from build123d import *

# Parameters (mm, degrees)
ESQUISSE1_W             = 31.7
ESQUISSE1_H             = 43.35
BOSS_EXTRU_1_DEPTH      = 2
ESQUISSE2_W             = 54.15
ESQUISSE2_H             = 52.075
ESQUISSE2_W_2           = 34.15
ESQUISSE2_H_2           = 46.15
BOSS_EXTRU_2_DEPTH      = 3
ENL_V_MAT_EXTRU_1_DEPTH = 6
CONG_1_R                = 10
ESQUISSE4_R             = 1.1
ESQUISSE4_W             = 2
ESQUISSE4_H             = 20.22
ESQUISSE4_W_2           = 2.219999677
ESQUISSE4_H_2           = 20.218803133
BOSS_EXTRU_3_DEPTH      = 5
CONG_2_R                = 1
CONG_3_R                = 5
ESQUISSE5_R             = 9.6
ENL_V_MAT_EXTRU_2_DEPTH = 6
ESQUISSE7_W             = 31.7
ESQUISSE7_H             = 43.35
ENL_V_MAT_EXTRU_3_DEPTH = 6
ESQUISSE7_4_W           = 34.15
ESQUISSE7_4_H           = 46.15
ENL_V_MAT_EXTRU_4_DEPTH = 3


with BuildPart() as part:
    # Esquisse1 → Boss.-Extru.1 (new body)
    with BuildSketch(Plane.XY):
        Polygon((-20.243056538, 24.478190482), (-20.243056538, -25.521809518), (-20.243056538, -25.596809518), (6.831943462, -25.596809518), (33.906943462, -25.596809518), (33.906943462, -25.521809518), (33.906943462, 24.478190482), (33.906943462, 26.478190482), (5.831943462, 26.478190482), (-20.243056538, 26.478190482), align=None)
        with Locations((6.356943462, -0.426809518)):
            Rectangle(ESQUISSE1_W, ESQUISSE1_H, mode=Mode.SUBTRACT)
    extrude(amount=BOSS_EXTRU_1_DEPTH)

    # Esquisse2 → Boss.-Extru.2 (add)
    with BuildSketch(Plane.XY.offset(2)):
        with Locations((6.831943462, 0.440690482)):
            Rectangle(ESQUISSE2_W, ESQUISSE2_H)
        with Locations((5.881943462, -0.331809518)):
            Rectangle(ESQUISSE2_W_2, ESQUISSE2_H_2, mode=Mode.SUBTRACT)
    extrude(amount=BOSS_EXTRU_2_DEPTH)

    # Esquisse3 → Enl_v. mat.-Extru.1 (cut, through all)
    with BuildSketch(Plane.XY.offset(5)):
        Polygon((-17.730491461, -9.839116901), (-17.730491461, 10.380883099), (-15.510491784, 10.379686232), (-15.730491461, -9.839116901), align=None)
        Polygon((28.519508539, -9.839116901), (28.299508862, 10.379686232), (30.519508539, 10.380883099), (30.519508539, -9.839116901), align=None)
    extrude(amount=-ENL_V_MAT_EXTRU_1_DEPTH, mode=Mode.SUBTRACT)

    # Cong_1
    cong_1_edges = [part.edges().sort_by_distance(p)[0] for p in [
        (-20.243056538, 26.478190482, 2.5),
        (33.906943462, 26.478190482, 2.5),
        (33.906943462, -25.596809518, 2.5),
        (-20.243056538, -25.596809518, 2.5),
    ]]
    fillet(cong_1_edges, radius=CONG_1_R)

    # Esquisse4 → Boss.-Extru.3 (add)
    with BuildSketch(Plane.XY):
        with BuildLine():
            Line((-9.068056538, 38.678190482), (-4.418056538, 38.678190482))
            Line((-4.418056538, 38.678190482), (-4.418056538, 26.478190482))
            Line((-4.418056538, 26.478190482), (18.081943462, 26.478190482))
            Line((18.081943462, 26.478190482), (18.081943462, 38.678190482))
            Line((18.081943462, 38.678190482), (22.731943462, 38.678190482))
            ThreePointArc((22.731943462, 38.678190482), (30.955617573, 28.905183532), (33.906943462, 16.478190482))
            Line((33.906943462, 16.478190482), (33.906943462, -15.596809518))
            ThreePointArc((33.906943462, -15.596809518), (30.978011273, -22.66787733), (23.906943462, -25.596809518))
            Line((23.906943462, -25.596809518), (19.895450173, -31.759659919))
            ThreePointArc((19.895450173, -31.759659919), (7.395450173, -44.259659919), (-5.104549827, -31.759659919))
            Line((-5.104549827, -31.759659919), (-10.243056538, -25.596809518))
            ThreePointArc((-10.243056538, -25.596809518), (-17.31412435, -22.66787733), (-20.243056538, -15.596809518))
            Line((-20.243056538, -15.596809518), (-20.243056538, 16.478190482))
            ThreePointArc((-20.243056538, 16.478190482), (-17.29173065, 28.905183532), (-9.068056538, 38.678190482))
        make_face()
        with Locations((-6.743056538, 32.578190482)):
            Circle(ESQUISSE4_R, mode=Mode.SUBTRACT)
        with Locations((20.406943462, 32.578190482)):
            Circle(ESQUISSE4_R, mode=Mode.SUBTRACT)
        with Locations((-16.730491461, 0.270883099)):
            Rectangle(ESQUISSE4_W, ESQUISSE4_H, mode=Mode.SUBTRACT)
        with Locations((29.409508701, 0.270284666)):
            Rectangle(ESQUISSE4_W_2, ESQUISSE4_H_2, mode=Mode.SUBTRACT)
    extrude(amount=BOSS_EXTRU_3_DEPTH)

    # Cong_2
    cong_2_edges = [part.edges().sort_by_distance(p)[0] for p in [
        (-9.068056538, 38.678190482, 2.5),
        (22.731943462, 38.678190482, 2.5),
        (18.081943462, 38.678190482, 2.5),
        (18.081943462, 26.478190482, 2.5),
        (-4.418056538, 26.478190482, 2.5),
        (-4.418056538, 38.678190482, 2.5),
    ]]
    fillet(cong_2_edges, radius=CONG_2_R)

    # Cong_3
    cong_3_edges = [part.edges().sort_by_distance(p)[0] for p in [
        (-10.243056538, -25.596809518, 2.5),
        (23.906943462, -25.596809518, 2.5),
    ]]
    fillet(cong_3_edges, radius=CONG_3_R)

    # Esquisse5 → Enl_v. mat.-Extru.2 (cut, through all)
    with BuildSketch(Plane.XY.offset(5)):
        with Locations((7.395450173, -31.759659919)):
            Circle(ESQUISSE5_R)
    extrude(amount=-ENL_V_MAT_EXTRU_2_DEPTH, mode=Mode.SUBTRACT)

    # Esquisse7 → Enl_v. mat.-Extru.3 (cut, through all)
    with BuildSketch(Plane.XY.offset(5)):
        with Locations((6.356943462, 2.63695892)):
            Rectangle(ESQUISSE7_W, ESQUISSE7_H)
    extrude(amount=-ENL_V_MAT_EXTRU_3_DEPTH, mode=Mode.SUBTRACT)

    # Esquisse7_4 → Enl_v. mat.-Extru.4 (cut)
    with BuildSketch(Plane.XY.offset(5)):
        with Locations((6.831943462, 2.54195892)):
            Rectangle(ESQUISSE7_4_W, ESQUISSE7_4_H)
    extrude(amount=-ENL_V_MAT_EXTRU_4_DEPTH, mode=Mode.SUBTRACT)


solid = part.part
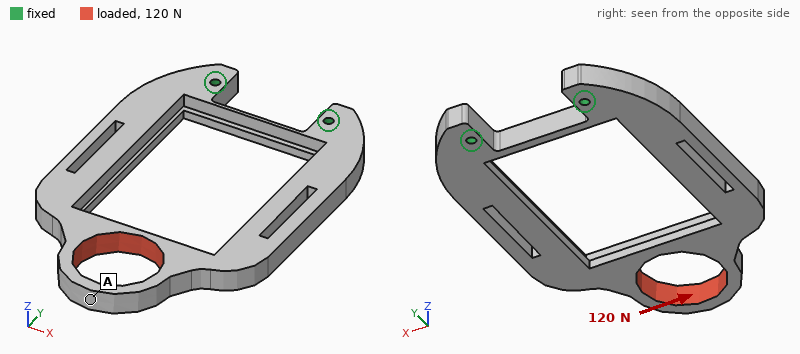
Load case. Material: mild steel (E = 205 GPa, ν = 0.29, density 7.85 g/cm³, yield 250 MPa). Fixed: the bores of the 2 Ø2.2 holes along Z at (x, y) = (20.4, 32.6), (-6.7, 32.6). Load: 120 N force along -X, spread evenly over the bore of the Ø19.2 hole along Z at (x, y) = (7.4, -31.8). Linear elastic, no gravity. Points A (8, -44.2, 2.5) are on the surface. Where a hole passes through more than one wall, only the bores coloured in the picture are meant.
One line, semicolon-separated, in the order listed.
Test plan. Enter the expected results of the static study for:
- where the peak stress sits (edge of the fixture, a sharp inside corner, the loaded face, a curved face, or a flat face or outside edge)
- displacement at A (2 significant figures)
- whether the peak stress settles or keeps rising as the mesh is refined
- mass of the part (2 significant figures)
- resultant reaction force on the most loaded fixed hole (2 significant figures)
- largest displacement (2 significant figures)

edge of the fixture; 50 µm; keeps rising; 62 g; 120 N; 51 µm
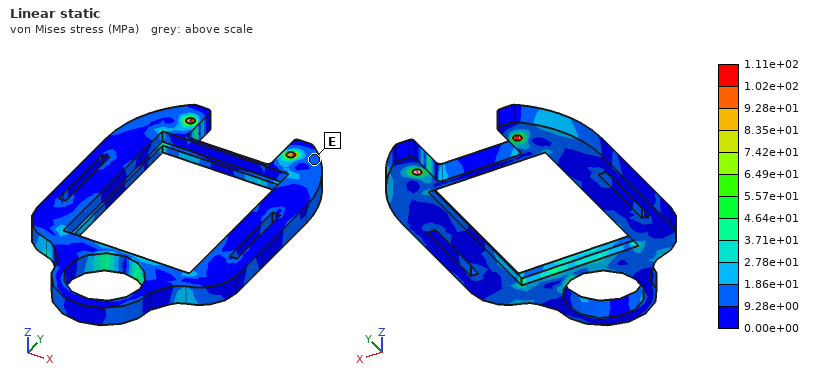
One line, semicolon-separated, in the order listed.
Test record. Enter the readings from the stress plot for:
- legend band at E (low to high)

9.28e+00 to 1.86e+01 MPa
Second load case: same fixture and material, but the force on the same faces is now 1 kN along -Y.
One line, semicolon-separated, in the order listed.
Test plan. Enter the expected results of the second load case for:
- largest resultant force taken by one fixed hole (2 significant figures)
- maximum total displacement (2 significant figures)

540 N; 28 µm
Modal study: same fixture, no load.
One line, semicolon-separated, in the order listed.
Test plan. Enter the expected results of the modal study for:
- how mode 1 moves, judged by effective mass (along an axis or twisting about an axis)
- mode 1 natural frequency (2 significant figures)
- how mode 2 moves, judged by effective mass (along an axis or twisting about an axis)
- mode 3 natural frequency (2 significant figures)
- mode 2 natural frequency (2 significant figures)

along Z; 730 Hz; along X; 1800 Hz; 1500 Hz
